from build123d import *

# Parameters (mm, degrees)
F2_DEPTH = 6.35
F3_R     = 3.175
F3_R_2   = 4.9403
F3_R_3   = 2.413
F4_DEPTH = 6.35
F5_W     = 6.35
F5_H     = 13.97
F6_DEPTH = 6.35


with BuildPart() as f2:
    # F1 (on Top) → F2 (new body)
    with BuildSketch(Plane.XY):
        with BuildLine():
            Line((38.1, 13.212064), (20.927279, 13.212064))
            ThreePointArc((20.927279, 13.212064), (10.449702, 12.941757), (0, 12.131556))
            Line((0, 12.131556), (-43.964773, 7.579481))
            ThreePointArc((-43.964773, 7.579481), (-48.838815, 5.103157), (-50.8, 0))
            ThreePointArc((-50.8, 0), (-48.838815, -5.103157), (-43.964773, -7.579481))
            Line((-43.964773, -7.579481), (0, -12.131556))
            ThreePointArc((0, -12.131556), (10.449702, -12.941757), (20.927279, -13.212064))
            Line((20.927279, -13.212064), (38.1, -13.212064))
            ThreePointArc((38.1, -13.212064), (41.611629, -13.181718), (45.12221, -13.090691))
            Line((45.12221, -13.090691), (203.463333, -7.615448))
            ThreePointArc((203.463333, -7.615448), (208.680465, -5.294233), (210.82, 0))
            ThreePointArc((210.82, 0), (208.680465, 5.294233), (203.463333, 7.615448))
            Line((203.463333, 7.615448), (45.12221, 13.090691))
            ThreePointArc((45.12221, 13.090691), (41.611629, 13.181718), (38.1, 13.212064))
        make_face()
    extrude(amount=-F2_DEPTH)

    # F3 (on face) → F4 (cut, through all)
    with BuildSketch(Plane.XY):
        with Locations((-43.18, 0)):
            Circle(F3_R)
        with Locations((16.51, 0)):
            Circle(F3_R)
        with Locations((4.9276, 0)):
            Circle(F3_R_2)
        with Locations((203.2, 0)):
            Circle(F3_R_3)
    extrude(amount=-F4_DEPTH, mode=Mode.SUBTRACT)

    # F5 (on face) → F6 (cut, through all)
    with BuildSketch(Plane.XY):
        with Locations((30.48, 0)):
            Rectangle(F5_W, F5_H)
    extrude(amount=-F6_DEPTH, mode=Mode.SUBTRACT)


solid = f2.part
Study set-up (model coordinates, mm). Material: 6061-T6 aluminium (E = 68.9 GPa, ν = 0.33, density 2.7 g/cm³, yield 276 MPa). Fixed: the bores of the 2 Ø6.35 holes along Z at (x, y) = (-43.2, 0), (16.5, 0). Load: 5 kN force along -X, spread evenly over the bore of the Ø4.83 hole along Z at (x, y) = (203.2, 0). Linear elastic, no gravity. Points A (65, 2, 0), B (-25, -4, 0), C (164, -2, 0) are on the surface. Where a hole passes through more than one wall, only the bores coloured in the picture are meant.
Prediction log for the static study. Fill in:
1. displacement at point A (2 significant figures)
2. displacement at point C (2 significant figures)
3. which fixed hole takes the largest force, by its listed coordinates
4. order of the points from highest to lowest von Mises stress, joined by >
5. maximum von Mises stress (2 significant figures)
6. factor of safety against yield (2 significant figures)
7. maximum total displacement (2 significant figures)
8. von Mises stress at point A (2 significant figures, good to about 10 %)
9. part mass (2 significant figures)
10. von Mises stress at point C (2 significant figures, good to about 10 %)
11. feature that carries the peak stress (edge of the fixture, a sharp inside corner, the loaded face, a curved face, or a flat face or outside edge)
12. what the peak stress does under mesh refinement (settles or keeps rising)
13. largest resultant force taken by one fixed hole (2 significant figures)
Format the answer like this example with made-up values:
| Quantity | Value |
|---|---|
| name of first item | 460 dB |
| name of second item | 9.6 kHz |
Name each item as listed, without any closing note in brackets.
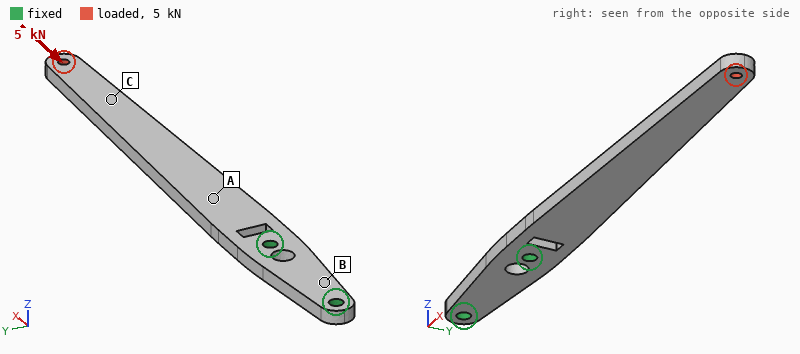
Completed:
| Quantity | Value |
|---|---|
| displacement at point A | 0.036 mm |
| displacement at point C | 0.089 mm |
| which fixed hole takes the largest force, by its listed coordinates | (16.5, 0) |
| order of the points from highest to lowest von Mises stress, joined by > | C > A > B |
| maximum von Mises stress | 140 MPa |
| factor of safety against yield | 2.0 |
| maximum total displacement | 0.12 mm |
| von Mises stress at point A | 31 MPa |
| part mass | 90 g |
| von Mises stress at point C | 44 MPa |
| feature that carries the peak stress | the loaded face |
| what the peak stress does under mesh refinement | settles |
| largest resultant force taken by one fixed hole | 4.3 kN |
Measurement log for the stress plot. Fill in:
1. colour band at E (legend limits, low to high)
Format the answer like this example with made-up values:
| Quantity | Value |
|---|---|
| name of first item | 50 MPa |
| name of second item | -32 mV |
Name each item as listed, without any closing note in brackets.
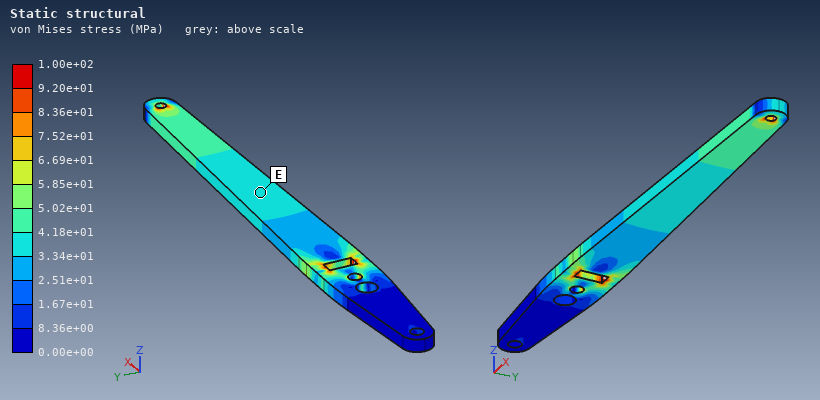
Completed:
| Quantity | Value |
|---|---|
| colour band at E | 3.34e+01 to 4.18e+01 MPa |
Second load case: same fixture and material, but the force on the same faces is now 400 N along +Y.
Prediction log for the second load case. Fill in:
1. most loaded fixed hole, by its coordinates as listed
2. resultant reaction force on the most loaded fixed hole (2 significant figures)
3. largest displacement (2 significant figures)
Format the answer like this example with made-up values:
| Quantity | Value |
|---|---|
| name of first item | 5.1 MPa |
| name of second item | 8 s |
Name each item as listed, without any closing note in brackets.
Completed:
| Quantity | Value |
|---|---|
| most loaded fixed hole, by its coordinates as listed | (16.5, 0) |
| resultant reaction force on the most loaded fixed hole | 1.2 kN |
| largest displacement | 2.2 mm |
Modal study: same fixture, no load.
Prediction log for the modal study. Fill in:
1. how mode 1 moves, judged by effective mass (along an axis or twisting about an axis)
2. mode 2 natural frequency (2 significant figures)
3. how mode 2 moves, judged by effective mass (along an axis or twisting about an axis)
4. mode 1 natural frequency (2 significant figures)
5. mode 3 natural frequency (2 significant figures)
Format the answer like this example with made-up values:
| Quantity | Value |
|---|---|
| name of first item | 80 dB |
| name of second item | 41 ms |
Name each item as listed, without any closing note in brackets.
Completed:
| Quantity | Value |
|---|---|
| how mode 1 moves, judged by effective mass | along Z |
| mode 2 natural frequency | 570 Hz |
| how mode 2 moves, judged by effective mass | along Y |
| mode 1 natural frequency | 150 Hz |
| mode 3 natural frequency | 880 Hz |
